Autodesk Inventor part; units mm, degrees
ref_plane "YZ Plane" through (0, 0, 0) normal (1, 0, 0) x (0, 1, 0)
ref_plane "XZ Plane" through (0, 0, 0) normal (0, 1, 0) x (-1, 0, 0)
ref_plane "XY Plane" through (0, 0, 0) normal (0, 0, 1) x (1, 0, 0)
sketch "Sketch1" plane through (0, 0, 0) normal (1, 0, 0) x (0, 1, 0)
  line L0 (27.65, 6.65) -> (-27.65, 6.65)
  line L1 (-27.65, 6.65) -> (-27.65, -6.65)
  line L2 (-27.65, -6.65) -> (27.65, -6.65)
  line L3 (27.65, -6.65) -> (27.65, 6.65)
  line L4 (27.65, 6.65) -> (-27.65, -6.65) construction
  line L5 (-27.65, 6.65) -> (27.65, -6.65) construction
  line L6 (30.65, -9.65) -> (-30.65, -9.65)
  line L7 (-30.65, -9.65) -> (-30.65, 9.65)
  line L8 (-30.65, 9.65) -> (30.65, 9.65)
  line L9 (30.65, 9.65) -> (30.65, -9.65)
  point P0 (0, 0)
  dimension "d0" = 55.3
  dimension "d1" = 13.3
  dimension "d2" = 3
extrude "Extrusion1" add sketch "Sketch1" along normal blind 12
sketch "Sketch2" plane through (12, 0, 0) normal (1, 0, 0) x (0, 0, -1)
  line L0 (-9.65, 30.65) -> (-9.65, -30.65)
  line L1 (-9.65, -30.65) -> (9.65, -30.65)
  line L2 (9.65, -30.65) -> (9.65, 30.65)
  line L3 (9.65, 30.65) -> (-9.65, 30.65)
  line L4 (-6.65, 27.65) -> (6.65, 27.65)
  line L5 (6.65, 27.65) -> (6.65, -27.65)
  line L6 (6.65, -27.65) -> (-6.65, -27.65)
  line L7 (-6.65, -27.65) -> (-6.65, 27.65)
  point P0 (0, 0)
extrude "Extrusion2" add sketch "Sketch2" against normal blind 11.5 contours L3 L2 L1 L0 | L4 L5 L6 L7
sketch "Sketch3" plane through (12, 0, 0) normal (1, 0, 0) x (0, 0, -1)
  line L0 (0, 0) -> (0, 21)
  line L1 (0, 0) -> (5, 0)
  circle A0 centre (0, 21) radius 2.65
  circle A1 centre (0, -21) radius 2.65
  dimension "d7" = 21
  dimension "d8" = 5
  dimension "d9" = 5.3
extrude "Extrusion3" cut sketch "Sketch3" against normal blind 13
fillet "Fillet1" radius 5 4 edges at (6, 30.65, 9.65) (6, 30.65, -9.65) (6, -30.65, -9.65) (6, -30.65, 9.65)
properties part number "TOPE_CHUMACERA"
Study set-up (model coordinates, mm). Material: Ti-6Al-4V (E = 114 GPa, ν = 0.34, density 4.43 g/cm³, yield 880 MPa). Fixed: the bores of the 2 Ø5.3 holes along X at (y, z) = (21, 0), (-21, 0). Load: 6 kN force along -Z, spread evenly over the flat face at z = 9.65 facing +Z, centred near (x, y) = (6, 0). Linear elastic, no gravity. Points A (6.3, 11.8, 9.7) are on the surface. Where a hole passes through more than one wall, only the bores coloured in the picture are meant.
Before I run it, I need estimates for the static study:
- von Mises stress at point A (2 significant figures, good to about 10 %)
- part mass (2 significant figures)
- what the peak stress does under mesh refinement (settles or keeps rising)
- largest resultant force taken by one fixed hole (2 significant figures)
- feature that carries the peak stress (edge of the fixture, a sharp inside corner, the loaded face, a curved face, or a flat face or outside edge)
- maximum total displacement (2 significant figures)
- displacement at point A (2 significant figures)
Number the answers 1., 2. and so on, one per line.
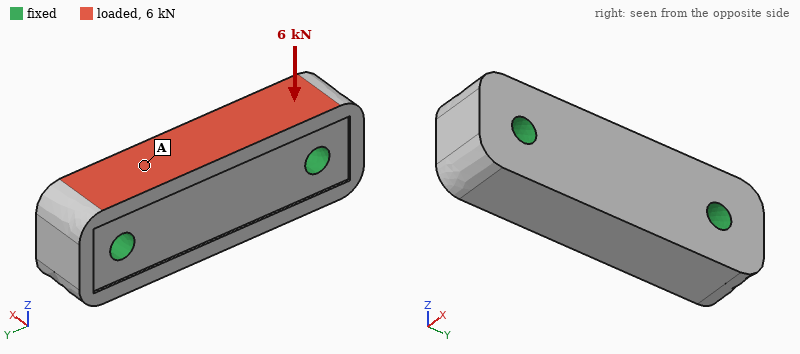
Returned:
1. 12 MPa
2. 58 g
3. keeps rising
4. 3.0 kN
5. edge of the fixture
6. 6.2 µm
7. 4.1 µm
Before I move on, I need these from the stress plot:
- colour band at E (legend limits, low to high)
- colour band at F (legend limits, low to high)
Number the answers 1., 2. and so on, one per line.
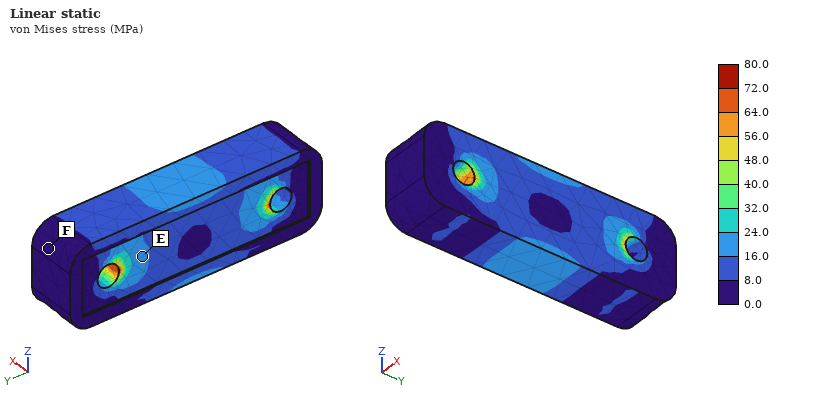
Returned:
1. 16.0 to 24.0 MPa
2. 0.0 to 8.0 MPa
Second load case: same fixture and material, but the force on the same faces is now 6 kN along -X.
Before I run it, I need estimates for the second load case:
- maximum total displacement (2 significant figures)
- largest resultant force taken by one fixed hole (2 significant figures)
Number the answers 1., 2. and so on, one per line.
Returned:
1. 20 µm
2. 3.0 kN
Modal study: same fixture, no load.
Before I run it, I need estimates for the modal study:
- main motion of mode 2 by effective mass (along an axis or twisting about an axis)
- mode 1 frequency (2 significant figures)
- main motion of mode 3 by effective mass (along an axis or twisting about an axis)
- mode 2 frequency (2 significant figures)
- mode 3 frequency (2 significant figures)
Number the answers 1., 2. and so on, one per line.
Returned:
1. along Z
2. 24 kHz
3. twisting about Y
4. 25 kHz
5. 30 kHz
